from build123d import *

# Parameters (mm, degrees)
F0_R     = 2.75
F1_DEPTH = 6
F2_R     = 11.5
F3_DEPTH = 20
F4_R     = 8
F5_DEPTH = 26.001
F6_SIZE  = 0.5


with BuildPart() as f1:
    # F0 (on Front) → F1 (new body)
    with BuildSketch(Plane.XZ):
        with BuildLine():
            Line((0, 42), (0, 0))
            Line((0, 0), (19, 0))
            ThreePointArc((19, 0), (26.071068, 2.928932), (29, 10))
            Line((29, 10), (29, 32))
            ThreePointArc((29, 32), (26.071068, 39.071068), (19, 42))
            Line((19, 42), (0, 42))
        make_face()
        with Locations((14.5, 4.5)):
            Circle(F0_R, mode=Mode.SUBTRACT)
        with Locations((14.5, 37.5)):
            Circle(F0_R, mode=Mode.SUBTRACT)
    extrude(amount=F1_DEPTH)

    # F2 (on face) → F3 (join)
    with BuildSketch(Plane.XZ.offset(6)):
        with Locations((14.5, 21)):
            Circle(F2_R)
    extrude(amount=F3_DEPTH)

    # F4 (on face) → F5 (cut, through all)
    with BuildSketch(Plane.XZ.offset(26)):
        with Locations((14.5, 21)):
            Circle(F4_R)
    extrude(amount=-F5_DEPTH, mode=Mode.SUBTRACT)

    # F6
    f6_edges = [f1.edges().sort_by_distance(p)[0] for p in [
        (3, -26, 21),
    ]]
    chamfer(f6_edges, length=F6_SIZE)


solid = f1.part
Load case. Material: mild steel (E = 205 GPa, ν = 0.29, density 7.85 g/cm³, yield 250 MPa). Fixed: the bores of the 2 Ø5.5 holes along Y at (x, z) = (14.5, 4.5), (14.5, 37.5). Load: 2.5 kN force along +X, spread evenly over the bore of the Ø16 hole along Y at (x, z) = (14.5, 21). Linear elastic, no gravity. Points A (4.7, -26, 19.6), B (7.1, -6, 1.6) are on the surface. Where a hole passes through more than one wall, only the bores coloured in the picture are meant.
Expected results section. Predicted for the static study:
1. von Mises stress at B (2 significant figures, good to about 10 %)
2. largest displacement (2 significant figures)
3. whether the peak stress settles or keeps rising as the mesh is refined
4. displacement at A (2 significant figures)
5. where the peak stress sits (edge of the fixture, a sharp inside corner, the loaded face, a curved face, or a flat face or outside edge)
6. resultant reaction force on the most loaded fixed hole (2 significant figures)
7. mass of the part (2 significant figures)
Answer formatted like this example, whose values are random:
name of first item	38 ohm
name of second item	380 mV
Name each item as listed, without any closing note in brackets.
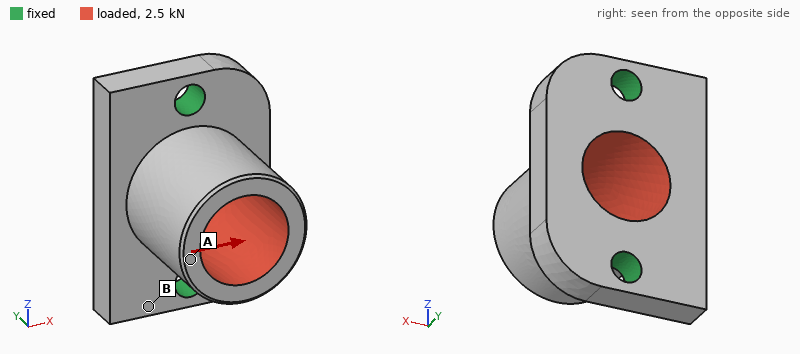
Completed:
von Mises stress at B	28 MPa
largest displacement	24 µm
whether the peak stress settles or keeps rising as the mesh is refined	keeps rising
displacement at A	24 µm
where the peak stress sits	edge of the fixture
resultant reaction force on the most loaded fixed hole	1.3 kN
mass of the part	77 g
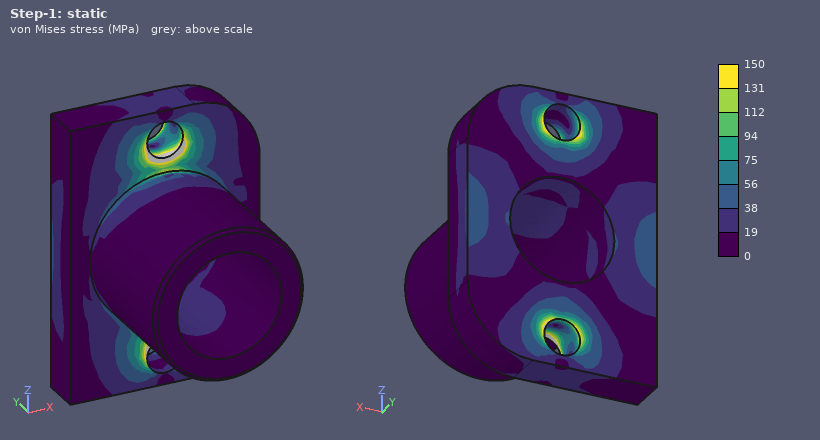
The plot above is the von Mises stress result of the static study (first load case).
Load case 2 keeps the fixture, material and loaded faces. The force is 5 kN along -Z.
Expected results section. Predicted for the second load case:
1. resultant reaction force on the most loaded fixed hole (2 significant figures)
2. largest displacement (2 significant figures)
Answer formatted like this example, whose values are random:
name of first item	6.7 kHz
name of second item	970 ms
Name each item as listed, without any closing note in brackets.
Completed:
resultant reaction force on the most loaded fixed hole	3.1 kN
largest displacement	12 µm
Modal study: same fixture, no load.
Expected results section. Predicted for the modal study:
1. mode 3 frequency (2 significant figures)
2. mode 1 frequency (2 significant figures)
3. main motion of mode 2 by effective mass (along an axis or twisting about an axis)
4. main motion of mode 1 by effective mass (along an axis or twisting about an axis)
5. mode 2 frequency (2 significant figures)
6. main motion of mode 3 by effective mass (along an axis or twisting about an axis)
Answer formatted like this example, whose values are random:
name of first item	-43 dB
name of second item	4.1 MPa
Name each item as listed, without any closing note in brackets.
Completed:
mode 3 frequency	19 kHz
mode 1 frequency	8200 Hz
main motion of mode 2 by effective mass	along Z
main motion of mode 1 by effective mass	along X
mode 2 frequency	18 kHz
main motion of mode 3 by effective mass	along Y
